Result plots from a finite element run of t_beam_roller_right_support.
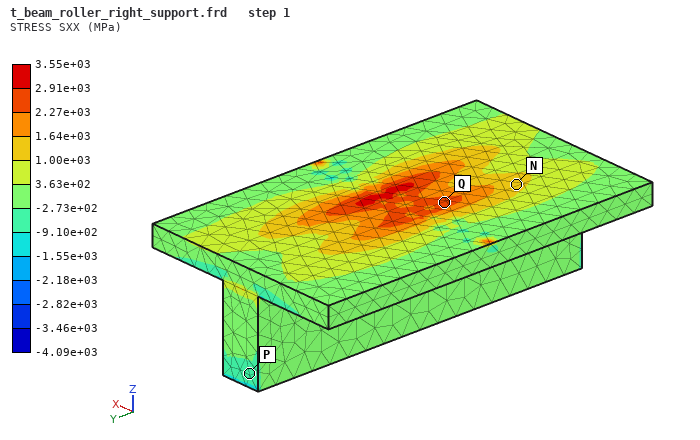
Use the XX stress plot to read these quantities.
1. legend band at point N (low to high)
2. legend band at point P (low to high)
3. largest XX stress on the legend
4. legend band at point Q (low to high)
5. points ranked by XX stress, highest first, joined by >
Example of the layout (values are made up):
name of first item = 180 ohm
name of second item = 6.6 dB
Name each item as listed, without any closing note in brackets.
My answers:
legend band at point N = 1.00e+03 to 1.64e+03 MPa
legend band at point P = -9.10e+02 to -2.73e+02 MPa
largest XX stress on the legend = 3.55e+03 MPa
legend band at point Q = 2.27e+03 to 2.91e+03 MPa
points ranked by XX stress, highest first, joined by > = Q > N > P
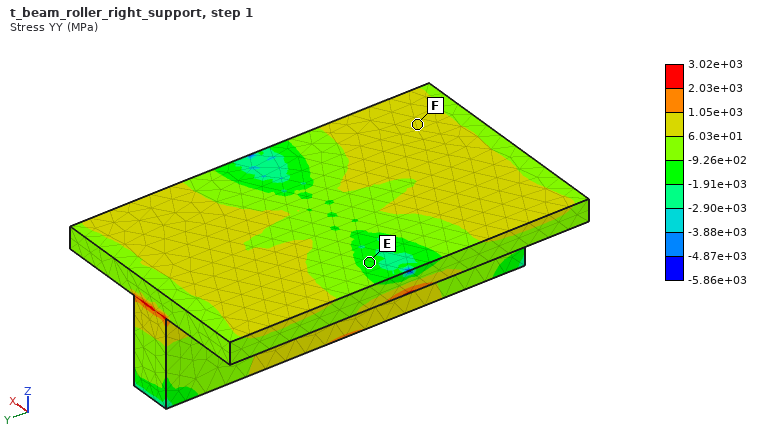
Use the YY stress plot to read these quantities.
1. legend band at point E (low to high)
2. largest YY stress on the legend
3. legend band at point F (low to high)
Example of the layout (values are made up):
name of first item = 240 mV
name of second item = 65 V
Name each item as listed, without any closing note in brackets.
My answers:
legend band at point E = -1.91e+03 to -9.26e+02 MPa
largest YY stress on the legend = 3.02e+03 MPa
legend band at point F = 6.03e+01 to 1.05e+03 MPa
